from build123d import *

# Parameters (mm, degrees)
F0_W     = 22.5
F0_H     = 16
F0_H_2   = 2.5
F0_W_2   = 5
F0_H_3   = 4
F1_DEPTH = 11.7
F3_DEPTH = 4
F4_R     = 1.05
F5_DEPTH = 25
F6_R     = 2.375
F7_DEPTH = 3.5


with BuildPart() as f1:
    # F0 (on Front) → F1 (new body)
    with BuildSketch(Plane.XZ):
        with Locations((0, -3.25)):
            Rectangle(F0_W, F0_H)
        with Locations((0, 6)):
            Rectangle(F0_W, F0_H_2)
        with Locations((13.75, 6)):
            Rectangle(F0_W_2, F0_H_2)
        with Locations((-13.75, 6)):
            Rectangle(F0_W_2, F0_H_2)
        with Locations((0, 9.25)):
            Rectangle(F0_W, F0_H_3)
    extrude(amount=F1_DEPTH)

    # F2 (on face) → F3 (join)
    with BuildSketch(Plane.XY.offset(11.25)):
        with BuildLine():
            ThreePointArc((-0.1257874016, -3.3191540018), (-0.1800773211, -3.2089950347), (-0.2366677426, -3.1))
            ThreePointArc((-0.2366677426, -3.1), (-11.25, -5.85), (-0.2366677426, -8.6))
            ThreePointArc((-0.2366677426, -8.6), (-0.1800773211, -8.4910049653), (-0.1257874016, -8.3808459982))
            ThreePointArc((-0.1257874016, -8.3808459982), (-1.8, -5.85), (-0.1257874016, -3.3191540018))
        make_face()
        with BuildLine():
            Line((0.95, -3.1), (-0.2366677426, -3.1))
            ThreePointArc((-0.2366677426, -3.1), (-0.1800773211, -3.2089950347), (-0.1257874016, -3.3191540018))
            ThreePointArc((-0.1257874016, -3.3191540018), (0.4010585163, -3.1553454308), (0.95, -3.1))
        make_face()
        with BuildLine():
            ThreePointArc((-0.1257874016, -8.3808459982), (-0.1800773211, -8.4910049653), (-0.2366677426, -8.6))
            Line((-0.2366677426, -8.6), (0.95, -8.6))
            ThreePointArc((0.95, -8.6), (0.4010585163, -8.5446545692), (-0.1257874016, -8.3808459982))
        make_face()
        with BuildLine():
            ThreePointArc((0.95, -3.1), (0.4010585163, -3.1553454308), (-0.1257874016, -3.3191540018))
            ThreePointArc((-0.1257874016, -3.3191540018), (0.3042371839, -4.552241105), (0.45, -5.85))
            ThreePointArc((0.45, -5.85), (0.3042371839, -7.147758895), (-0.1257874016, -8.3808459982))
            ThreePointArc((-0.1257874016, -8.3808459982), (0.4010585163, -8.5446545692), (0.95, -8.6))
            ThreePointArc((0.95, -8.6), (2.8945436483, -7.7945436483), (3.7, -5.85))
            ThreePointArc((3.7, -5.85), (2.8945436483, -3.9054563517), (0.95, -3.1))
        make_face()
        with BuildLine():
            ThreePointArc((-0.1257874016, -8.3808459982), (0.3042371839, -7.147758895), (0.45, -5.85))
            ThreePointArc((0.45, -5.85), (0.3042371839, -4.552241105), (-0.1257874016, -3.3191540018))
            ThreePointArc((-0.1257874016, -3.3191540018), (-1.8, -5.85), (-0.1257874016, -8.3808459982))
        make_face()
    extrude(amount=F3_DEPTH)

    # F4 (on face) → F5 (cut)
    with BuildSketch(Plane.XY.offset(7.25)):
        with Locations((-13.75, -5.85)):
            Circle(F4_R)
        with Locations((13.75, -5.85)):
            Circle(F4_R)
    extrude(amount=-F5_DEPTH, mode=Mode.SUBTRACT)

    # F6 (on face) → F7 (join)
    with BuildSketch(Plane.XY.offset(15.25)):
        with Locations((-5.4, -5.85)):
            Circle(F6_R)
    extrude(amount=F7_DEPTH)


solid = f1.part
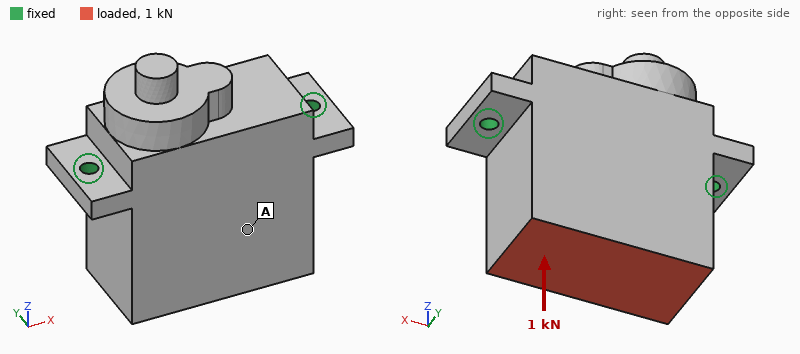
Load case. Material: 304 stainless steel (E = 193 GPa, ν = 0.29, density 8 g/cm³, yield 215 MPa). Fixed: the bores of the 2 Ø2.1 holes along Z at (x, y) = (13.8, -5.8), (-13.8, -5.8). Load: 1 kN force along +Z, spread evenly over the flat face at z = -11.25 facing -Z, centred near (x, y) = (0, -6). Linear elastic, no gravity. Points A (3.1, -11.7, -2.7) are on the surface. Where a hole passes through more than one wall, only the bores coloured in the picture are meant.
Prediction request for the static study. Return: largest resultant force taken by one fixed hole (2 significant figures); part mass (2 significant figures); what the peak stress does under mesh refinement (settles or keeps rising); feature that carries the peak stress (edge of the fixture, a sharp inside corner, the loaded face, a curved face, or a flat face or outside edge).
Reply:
500 N
54 g
keeps rising
edge of the fixture
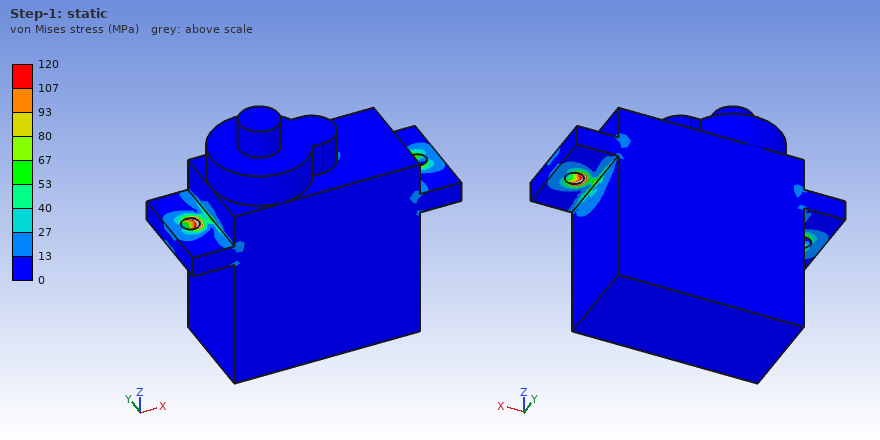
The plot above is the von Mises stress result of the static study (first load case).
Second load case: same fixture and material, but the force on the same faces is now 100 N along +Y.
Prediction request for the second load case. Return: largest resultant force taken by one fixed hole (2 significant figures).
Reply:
50 N
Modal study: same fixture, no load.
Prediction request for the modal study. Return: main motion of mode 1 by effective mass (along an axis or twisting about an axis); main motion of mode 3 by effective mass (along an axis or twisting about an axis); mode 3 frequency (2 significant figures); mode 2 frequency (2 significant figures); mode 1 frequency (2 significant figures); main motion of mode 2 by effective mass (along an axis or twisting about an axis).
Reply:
along Y
along X
16 kHz
15 kHz
3900 Hz
along Z
